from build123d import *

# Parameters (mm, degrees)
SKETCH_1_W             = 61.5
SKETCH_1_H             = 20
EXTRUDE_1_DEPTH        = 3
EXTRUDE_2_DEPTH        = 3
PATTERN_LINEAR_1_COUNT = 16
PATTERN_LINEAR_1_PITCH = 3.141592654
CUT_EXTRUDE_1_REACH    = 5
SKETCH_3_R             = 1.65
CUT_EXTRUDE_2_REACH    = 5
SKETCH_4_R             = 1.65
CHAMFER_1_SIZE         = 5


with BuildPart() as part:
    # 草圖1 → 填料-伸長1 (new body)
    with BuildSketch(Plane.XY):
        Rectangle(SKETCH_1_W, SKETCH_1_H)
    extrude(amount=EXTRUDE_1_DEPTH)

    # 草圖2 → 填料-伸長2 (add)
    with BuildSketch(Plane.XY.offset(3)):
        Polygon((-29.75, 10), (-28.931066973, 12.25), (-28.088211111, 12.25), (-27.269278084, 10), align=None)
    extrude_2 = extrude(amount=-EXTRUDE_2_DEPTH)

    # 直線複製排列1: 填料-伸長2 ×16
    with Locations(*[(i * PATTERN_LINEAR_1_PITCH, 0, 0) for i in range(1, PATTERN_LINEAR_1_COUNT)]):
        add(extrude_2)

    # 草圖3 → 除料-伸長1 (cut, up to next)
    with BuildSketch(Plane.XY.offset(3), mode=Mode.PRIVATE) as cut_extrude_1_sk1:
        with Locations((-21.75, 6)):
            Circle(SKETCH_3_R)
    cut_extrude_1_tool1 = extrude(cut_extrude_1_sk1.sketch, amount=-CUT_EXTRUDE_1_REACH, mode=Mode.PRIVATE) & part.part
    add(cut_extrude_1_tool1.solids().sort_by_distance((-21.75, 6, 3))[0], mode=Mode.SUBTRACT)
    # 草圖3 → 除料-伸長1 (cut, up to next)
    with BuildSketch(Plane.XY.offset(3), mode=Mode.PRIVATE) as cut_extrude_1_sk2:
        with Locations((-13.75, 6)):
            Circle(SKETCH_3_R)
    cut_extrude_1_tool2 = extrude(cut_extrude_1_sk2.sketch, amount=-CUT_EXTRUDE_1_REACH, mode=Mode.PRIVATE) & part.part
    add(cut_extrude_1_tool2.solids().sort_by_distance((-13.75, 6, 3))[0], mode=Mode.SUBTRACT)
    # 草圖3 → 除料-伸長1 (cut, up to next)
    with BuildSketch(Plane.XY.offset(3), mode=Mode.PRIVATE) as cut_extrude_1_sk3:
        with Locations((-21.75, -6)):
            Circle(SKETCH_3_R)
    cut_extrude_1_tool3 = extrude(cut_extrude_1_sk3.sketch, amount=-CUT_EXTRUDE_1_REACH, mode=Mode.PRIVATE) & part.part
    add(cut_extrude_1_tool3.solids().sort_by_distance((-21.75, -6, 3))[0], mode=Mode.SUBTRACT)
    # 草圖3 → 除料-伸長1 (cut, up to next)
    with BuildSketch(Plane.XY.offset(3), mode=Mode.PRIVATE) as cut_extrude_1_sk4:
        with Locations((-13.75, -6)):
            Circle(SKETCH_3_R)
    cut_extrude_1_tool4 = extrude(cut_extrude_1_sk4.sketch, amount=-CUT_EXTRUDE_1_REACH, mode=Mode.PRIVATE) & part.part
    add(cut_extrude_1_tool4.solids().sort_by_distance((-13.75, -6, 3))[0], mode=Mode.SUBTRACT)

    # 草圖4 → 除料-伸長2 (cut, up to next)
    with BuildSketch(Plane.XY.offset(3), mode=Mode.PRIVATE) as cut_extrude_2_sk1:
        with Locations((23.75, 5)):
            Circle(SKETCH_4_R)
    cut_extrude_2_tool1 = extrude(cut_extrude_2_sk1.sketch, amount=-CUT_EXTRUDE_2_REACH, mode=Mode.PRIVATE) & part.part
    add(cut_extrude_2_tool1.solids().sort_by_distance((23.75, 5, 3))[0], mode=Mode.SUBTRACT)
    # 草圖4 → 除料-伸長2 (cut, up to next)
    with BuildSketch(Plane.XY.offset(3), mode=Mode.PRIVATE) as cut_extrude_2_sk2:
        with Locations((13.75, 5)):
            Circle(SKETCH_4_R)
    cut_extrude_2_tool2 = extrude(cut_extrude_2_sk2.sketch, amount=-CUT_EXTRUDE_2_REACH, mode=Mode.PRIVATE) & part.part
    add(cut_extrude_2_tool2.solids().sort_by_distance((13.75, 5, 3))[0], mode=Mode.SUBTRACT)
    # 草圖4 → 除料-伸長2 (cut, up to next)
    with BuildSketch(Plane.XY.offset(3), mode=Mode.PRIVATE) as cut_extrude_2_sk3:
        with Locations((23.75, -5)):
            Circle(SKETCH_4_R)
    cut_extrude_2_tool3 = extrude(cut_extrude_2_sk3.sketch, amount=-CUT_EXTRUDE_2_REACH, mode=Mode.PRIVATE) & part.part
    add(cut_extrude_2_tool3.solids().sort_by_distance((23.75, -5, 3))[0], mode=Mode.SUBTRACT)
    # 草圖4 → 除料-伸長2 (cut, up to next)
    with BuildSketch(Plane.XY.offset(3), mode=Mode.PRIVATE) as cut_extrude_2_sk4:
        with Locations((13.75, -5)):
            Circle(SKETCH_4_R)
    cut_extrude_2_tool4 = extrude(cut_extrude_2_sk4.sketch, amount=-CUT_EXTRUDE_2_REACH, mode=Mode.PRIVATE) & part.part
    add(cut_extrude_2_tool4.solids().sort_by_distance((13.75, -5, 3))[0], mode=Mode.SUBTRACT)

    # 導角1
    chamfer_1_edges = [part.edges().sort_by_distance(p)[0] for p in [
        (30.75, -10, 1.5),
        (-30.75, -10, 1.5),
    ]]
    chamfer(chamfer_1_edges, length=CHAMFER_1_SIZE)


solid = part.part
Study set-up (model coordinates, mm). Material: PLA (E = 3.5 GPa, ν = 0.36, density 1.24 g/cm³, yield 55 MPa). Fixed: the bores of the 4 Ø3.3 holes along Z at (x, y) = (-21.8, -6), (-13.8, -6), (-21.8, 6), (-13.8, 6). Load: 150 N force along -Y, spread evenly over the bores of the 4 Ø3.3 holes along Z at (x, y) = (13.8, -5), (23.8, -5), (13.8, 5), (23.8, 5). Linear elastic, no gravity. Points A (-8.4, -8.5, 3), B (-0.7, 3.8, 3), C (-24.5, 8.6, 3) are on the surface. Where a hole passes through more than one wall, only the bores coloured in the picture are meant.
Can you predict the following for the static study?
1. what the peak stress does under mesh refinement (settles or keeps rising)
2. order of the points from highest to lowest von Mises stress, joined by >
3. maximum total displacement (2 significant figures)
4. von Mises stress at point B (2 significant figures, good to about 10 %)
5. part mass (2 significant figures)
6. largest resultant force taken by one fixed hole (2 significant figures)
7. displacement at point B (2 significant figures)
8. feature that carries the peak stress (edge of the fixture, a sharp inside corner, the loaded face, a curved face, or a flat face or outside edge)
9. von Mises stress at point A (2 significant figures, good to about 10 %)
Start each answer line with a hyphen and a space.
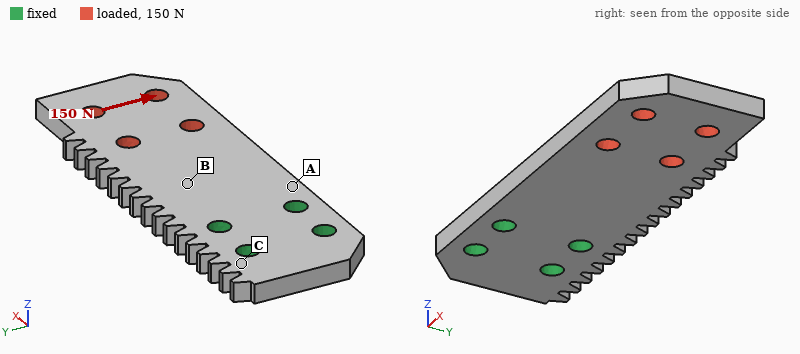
- keeps rising
- A > B > C
- 0.48 mm
- 7.8 MPa
- 4.5 g
- 320 N
- 0.082 mm
- edge of the fixture
- 16 MPa
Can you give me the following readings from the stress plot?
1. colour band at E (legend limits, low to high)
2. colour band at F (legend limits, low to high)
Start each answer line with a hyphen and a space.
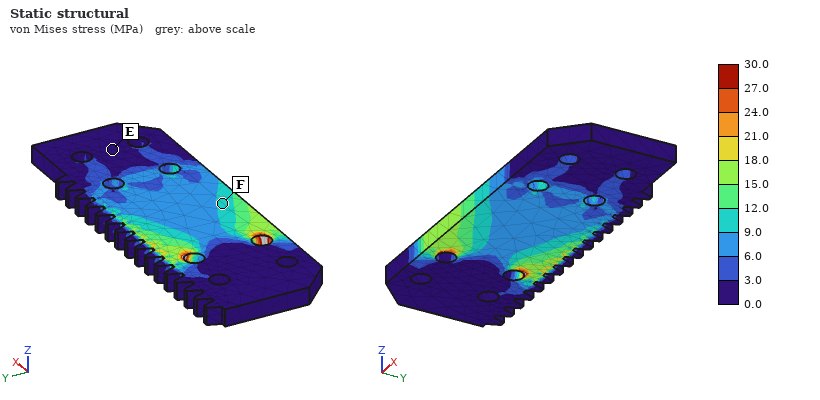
- 0.0 to 3.0 MPa
- 9.0 to 12.0 MPa
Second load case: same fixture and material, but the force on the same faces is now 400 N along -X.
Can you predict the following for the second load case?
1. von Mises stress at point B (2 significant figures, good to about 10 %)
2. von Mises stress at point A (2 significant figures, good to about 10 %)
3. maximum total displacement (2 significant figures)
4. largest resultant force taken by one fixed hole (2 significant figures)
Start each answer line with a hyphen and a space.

- 6.6 MPa
- 6.7 MPa
- 71 µm
- 180 N
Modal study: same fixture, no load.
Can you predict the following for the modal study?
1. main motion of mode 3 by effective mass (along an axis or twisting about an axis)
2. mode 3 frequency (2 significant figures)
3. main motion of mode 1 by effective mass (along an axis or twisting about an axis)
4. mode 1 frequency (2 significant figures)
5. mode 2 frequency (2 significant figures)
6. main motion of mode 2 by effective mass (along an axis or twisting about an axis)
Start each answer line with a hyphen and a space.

- along Y
- 2500 Hz
- along Z
- 450 Hz
- 1900 Hz
- twisting about X
